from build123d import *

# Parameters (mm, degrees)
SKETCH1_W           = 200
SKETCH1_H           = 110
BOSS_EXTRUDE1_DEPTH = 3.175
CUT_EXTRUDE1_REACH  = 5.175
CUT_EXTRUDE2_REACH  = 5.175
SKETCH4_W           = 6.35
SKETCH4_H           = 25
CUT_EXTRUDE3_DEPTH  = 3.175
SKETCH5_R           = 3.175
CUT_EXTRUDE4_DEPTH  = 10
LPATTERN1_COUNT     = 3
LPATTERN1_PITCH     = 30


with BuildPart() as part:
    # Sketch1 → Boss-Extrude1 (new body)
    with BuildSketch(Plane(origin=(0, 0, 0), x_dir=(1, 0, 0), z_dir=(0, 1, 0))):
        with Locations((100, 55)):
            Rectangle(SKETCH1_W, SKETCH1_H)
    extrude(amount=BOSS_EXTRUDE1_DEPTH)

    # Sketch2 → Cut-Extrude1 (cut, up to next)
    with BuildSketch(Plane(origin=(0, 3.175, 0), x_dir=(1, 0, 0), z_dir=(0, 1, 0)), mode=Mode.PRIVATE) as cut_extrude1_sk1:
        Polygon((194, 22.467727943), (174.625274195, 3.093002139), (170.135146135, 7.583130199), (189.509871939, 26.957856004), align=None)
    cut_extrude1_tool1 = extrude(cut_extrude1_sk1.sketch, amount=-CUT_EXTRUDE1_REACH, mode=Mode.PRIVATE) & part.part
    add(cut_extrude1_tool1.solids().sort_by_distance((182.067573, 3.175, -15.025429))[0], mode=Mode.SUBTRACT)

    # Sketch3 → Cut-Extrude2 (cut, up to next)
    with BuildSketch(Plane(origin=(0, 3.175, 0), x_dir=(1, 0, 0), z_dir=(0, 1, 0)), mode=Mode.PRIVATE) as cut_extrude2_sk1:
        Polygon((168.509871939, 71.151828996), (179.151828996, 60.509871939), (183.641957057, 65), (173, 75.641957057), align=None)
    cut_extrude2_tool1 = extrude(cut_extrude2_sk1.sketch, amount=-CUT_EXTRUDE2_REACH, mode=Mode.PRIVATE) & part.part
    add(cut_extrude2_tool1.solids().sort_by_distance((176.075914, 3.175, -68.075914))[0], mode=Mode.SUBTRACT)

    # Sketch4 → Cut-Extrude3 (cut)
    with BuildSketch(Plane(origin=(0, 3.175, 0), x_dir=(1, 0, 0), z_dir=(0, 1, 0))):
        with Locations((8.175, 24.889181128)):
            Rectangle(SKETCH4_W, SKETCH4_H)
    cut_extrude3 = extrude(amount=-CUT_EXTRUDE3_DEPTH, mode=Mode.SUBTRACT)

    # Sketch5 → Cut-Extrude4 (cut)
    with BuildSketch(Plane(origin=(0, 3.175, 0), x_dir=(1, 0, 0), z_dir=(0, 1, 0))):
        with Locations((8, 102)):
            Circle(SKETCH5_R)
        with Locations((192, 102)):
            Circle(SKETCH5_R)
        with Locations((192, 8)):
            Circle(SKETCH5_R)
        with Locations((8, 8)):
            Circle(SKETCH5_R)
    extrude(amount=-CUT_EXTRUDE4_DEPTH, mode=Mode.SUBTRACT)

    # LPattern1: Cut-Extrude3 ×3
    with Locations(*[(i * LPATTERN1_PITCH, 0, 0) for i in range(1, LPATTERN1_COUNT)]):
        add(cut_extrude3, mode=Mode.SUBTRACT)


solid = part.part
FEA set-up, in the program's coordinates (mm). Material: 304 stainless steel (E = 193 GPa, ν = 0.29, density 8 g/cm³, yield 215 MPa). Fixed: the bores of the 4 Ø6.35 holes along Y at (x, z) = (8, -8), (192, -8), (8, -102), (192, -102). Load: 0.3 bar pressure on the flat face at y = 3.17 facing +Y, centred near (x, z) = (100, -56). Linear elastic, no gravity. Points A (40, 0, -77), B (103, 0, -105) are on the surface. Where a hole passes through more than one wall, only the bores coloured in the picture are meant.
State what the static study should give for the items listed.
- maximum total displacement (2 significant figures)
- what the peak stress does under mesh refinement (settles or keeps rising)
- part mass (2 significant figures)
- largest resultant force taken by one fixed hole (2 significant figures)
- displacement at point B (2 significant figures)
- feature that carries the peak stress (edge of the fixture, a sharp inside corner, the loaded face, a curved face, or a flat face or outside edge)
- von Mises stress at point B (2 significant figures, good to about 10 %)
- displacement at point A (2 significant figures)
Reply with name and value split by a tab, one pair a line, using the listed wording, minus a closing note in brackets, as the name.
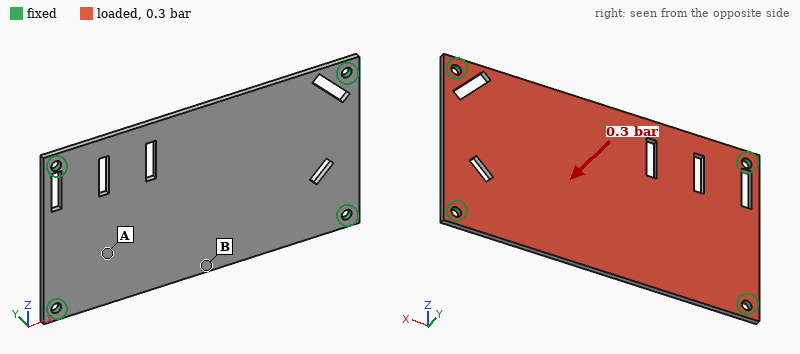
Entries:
maximum total displacement	0.28 mm
what the peak stress does under mesh refinement	keeps rising
part mass	540 g
largest resultant force taken by one fixed hole	180 N
displacement at point B	0.24 mm
feature that carries the peak stress	edge of the fixture
von Mises stress at point B	33 MPa
displacement at point A	0.11 mm
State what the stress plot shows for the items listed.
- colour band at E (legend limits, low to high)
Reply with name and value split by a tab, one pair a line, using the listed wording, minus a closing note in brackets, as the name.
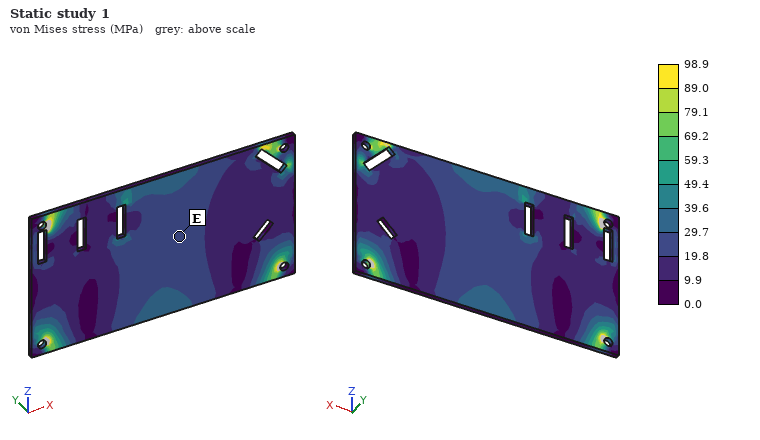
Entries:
colour band at E	19.8 to 29.7 MPa
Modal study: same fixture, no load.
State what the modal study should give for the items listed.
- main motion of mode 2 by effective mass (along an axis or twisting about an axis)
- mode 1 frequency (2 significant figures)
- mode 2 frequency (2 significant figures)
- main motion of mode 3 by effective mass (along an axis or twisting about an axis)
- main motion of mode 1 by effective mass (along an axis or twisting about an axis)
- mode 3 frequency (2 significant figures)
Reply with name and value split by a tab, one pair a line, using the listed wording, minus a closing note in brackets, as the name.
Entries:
main motion of mode 2 by effective mass	twisting about X
mode 1 frequency	380 Hz
mode 2 frequency	690 Hz
main motion of mode 3 by effective mass	twisting about Z
main motion of mode 1 by effective mass	along Y
mode 3 frequency	1000 Hz
